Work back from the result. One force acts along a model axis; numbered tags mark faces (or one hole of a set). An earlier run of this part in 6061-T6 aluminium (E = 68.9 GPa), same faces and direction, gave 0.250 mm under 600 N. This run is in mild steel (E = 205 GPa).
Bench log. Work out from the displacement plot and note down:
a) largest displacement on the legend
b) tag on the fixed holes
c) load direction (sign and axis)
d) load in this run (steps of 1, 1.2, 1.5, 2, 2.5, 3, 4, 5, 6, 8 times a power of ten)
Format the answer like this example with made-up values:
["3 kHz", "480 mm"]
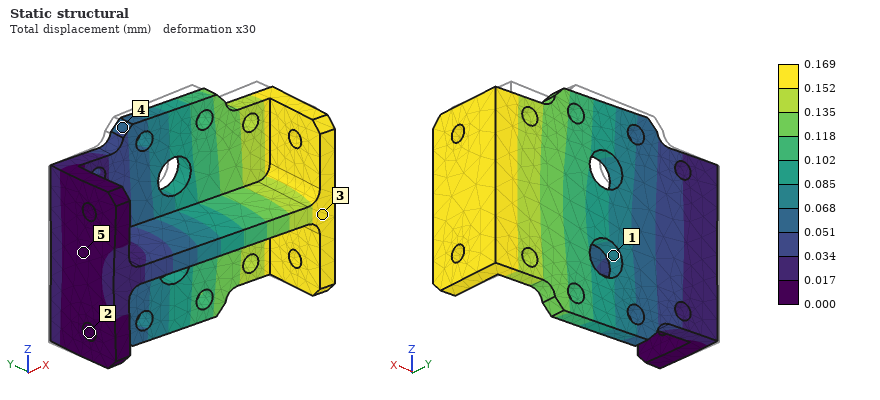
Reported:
["0.169 mm", "2", "-Y", "1.2 kN"]
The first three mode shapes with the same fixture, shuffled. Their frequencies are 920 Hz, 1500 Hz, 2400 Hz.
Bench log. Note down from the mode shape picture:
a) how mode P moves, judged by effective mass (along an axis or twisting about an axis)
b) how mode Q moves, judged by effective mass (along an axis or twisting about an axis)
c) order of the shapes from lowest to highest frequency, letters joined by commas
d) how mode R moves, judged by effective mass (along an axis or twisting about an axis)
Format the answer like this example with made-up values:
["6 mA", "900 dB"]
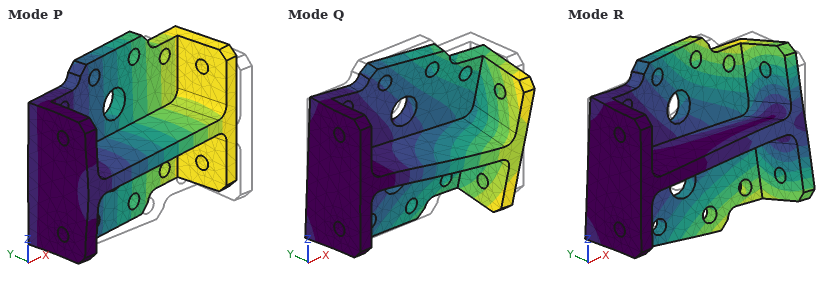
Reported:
["along Y", "along Z", "P, Q, R", "along Z"]
